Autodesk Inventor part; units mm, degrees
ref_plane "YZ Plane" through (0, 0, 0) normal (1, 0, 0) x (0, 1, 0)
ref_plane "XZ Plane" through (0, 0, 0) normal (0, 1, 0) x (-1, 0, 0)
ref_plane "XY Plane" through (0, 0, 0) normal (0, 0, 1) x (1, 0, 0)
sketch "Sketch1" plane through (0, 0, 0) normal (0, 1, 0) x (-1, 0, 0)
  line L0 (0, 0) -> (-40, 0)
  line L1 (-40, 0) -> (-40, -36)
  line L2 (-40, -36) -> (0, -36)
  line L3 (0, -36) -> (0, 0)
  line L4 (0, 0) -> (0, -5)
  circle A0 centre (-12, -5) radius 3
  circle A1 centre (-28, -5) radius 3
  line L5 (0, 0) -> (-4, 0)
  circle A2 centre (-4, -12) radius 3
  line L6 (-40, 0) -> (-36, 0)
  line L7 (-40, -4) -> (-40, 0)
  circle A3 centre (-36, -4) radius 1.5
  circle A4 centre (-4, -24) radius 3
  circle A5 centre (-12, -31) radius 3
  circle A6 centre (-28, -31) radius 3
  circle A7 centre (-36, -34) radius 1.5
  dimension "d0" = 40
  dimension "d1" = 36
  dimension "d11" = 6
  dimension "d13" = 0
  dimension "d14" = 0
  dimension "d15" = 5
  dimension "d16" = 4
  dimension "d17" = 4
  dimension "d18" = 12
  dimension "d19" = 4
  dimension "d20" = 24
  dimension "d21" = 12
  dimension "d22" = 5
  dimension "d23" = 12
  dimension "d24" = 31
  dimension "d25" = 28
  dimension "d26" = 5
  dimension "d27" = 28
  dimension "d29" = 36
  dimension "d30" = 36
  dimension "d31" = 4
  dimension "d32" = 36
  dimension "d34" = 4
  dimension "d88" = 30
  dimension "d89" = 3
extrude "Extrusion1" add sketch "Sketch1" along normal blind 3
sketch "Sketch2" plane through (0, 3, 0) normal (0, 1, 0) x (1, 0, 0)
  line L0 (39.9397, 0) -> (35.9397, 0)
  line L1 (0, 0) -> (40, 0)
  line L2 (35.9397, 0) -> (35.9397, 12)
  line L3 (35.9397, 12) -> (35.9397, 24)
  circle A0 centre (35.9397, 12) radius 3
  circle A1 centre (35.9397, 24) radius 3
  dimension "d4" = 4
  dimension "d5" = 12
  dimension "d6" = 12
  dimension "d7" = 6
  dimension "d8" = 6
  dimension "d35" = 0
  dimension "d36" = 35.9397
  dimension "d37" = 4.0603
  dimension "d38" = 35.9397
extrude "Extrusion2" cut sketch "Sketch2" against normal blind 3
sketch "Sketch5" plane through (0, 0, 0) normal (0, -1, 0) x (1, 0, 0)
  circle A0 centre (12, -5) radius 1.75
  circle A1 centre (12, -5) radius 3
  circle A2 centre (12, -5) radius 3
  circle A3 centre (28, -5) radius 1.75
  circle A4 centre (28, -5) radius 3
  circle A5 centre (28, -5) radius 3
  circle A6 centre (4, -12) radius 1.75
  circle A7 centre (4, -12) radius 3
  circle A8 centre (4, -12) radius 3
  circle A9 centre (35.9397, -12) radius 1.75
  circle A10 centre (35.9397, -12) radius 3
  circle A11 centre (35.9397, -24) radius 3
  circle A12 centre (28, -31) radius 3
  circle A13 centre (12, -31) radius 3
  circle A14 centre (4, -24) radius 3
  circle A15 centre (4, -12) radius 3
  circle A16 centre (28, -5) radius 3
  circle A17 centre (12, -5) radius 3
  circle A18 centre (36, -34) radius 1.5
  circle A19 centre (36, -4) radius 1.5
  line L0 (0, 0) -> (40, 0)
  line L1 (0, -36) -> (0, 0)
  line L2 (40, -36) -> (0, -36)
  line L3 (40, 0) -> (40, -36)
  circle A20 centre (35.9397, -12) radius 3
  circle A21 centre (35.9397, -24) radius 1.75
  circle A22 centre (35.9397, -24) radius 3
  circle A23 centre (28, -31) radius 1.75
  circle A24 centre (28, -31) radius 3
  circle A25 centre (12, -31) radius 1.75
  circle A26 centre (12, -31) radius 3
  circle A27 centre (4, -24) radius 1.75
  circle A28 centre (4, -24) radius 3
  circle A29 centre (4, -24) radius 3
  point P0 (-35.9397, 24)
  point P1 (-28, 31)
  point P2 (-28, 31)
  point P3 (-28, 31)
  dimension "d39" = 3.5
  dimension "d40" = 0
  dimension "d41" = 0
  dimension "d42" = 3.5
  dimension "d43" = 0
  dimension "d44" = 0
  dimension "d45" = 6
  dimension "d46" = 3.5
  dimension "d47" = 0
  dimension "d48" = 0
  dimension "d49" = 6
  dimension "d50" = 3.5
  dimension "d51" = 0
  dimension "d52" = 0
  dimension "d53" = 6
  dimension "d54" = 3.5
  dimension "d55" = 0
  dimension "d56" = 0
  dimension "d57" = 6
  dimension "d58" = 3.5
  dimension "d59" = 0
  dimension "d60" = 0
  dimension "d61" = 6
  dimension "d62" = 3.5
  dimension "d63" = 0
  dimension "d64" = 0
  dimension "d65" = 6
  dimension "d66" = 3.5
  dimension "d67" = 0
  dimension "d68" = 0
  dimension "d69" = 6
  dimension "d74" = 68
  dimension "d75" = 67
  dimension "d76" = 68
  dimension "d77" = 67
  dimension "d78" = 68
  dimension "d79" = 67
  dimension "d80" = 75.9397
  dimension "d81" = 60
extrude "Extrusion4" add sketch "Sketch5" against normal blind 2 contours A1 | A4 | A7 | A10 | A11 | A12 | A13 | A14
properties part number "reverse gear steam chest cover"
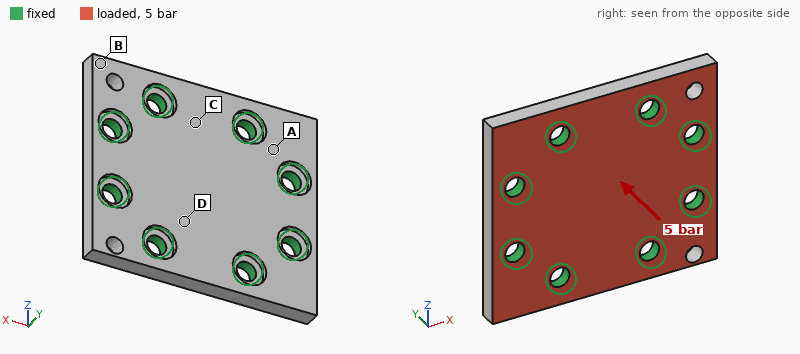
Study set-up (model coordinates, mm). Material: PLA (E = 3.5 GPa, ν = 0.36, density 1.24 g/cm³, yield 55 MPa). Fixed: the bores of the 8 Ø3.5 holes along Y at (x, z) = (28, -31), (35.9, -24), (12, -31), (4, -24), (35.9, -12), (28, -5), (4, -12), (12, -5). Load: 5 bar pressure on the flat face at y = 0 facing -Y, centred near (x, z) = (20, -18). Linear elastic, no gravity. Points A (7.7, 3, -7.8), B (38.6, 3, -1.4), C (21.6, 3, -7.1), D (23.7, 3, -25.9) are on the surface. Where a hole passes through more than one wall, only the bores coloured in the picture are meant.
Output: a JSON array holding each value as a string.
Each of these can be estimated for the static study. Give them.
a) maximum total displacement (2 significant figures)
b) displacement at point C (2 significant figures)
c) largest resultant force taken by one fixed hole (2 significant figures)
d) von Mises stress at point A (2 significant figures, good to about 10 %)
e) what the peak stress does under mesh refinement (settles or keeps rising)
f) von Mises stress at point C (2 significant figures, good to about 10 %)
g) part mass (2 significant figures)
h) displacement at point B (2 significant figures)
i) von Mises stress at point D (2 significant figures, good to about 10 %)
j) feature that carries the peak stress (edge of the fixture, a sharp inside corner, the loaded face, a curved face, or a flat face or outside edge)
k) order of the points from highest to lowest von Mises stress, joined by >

["70 µm", "28 µm", "100 N", "8.6 MPa", "keeps rising", "5.7 MPa", "4.8 g", "53 µm", "3.6 MPa", "edge of the fixture", "A > C > D > B"]
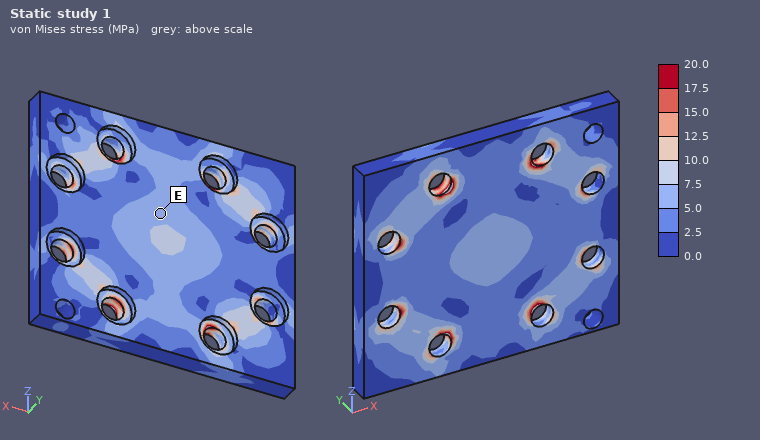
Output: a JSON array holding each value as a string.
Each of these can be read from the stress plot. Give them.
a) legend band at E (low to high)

["5.0 to 7.5 MPa"]
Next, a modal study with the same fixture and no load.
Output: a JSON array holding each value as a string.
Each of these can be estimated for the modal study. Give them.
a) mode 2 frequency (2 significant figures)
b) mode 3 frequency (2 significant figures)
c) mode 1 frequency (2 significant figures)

["9000 Hz", "9000 Hz", "8100 Hz"]
